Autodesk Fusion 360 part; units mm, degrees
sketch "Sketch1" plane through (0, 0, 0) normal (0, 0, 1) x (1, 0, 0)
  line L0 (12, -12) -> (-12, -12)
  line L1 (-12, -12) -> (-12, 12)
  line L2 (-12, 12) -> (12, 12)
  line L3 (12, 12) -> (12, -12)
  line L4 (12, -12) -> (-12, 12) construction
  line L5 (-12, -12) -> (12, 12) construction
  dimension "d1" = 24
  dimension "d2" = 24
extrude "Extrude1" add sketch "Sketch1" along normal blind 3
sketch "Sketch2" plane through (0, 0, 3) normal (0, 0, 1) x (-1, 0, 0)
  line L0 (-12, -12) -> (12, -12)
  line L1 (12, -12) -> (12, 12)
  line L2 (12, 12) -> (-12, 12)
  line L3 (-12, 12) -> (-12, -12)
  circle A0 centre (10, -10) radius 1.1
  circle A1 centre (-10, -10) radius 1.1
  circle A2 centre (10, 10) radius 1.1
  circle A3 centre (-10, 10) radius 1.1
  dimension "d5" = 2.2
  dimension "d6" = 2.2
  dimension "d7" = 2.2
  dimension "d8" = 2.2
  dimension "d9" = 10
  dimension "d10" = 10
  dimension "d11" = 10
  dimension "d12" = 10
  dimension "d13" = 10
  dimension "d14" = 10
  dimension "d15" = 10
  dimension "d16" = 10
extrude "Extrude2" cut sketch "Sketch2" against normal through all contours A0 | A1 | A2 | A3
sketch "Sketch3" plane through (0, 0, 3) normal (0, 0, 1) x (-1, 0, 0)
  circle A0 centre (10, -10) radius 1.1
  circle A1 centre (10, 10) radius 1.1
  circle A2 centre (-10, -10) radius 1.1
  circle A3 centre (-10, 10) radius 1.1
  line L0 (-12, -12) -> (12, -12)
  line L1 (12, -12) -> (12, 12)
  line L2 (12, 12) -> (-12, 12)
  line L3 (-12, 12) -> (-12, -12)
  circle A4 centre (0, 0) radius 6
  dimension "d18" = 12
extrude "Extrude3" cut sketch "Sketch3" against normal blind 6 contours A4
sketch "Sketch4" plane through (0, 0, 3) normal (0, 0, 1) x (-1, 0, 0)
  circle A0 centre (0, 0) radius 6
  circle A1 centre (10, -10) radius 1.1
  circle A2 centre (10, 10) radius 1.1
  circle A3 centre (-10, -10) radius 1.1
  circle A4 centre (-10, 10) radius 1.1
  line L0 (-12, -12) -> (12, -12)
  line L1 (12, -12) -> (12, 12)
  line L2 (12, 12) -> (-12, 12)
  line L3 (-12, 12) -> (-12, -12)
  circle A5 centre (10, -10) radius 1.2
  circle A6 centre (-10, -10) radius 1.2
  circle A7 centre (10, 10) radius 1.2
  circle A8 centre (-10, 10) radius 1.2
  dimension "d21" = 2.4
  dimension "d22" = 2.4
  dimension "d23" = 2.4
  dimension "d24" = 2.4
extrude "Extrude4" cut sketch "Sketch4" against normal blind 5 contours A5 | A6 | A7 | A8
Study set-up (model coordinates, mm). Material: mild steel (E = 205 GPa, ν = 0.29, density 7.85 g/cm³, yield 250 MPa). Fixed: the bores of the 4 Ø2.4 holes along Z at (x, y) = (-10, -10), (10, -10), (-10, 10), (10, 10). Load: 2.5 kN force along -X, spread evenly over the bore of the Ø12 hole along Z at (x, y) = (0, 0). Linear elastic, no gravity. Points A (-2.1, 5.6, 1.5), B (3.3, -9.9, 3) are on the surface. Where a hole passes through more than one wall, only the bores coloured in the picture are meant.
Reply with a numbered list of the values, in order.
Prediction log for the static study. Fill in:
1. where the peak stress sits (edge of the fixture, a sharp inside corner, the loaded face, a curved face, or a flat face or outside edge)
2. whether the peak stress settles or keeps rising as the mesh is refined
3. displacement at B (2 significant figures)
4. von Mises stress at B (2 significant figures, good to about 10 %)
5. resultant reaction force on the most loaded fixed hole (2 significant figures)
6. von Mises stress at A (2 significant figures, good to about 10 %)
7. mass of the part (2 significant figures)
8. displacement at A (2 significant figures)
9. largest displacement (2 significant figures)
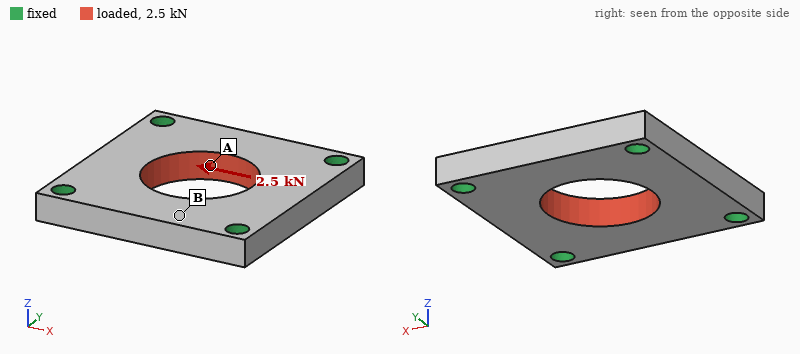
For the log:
1. edge of the fixture
2. keeps rising
3. 0.82 µm
4. 22 MPa
5. 670 N
6. 46 MPa
7. 10 g
8. 1.6 µm
9. 2.8 µm
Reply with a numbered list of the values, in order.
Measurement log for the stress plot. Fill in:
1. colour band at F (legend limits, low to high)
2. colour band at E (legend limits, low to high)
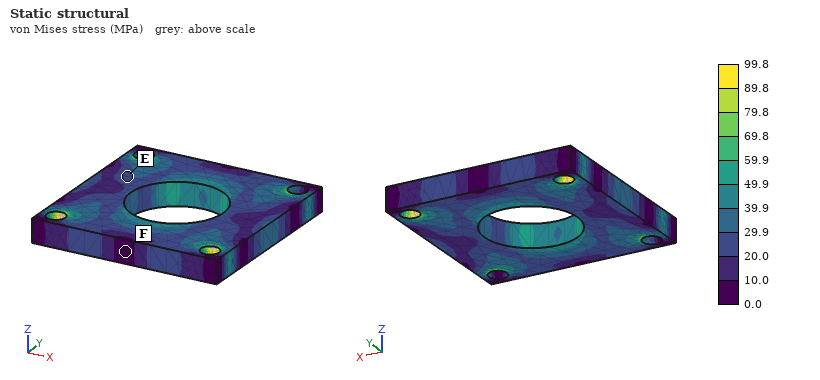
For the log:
1. 0.0 to 10.0 MPa
2. 20.0 to 29.9 MPa
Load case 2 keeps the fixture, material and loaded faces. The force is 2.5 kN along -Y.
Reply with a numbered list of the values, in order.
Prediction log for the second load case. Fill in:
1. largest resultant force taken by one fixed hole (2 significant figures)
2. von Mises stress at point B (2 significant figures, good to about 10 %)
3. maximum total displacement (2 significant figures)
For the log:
1. 670 N
2. 20 MPa
3. 2.8 µm
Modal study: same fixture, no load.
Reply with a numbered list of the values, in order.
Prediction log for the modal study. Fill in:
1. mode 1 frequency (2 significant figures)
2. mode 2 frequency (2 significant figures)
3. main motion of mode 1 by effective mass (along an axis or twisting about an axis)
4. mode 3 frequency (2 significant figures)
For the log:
1. 31 kHz
2. 39 kHz
3. along Z
4. 39 kHz
